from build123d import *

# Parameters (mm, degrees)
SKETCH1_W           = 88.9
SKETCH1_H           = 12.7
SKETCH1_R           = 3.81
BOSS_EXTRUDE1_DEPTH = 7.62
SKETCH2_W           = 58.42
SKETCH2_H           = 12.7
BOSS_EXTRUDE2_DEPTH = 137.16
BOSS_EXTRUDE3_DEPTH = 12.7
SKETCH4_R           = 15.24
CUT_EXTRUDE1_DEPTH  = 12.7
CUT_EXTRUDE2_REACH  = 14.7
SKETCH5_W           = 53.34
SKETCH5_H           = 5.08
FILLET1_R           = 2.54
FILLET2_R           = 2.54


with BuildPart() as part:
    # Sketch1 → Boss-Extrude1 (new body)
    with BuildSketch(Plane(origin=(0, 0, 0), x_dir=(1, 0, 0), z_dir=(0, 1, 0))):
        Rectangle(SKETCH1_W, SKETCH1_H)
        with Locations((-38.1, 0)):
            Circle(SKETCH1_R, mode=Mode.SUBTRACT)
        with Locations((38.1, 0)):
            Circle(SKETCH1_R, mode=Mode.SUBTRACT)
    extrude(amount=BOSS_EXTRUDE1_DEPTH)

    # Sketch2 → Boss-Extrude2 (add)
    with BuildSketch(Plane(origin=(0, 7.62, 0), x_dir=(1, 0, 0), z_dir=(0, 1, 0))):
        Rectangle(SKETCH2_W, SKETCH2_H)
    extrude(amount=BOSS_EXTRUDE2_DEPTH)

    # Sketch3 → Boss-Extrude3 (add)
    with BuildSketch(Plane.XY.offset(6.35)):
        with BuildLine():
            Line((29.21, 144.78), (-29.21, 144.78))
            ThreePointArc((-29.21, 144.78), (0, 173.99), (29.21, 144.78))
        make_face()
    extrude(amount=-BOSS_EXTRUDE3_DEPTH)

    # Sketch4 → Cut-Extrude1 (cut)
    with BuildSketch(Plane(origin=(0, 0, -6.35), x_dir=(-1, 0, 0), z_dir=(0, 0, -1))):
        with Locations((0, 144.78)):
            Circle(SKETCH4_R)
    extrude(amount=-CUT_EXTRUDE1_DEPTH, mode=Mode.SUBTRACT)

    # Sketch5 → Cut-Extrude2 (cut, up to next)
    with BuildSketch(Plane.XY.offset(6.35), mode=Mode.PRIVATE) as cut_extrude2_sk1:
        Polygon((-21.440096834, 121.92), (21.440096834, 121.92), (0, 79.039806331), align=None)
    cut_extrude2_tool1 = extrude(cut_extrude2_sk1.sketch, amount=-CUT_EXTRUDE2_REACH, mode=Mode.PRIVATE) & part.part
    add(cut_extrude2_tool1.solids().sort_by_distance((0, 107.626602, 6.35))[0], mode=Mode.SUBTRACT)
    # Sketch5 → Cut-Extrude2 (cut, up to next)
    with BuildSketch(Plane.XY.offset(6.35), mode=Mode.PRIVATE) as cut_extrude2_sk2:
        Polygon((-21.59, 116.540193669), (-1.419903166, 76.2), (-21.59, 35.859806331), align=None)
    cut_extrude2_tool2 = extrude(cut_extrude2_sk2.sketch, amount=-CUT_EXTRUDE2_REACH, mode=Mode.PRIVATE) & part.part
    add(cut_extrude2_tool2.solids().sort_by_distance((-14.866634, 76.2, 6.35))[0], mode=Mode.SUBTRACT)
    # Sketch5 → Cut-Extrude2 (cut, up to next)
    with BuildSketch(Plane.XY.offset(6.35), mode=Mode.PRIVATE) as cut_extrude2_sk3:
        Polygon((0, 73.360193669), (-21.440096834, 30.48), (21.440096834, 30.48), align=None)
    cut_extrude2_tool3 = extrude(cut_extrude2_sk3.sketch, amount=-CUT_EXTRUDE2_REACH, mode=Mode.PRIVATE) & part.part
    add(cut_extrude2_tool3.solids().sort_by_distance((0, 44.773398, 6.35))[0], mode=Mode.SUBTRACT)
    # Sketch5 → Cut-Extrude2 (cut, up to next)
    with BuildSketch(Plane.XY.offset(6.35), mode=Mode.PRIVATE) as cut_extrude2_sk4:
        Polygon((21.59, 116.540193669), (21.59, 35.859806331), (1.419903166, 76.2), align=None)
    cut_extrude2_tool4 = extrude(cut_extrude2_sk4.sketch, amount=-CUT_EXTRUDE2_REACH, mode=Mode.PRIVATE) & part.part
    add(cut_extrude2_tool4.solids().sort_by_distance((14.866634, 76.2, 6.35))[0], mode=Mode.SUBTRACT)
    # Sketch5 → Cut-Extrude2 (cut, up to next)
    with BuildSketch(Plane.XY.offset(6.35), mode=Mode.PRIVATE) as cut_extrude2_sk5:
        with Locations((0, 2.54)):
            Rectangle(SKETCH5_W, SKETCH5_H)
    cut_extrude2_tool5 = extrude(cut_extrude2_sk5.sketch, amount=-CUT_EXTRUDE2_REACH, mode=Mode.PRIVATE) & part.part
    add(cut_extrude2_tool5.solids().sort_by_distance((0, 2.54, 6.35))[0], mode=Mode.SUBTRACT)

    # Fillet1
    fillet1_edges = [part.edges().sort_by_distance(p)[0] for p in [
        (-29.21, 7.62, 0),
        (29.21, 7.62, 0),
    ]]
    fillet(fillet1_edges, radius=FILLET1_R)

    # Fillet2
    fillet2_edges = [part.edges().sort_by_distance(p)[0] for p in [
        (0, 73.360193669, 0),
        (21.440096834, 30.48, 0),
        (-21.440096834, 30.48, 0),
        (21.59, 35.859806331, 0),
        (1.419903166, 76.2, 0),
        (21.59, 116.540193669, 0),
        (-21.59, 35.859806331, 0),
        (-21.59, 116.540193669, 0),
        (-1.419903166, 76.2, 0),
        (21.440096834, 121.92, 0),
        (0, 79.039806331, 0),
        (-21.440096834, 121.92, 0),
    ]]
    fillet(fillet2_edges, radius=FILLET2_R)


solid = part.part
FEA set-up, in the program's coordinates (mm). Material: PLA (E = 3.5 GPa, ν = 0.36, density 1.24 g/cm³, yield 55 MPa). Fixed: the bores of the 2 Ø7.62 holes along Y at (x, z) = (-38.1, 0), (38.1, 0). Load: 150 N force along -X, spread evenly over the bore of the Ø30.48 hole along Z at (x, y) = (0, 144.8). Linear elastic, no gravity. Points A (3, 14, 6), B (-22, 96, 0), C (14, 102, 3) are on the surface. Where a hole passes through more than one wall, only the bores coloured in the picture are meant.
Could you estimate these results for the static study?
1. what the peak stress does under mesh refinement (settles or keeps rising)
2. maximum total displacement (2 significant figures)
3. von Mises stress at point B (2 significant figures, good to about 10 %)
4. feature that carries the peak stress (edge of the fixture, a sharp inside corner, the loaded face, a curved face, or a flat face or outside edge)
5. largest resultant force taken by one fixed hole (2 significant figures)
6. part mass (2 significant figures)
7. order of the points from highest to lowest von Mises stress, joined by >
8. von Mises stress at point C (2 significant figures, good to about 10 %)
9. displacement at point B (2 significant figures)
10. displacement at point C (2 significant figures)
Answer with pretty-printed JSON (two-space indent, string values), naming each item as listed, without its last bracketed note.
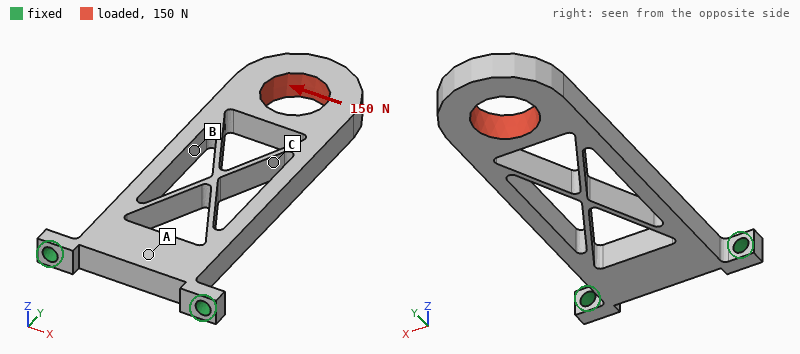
{
  "what the peak stress does under mesh refinement": "keeps rising",
  "maximum total displacement": "0.88 mm",
  "von Mises stress at point B": "3.5 MPa",
  "feature that carries the peak stress": "edge of the fixture",
  "largest resultant force taken by one fixed hole": "360 N",
  "part mass": "88 g",
  "order of the points from highest to lowest von Mises stress, joined by >": "C > B > A",
  "von Mises stress at point C": "5.8 MPa",
  "displacement at point B": "0.47 mm",
  "displacement at point C": "0.52 mm"
}
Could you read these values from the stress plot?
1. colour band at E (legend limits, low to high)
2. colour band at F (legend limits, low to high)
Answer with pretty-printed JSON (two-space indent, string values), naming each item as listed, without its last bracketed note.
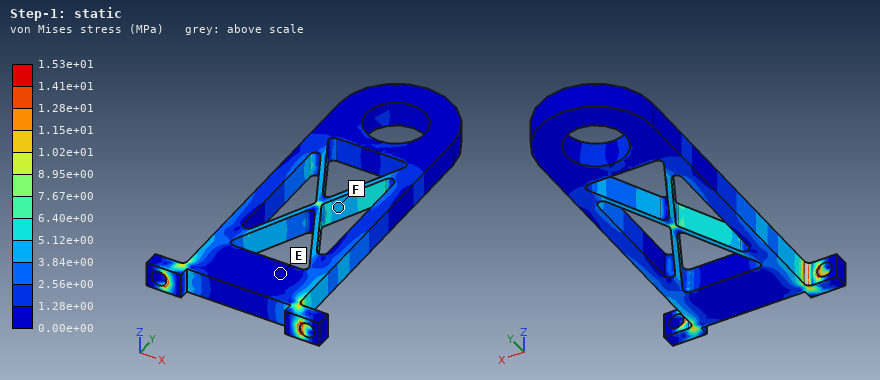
{
  "colour band at E": "0.00e+00 to 1.28e+00 MPa",
  "colour band at F": "3.84e+00 to 5.12e+00 MPa"
}
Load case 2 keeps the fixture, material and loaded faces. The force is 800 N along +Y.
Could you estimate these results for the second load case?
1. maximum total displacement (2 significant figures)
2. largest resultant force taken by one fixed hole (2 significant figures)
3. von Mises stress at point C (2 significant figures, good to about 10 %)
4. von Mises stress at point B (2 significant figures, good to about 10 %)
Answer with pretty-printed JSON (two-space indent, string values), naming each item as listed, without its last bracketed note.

{
  "maximum total displacement": "0.20 mm",
  "largest resultant force taken by one fixed hole": "460 N",
  "von Mises stress at point C": "1.4 MPa",
  "von Mises stress at point B": "4.5 MPa"
}
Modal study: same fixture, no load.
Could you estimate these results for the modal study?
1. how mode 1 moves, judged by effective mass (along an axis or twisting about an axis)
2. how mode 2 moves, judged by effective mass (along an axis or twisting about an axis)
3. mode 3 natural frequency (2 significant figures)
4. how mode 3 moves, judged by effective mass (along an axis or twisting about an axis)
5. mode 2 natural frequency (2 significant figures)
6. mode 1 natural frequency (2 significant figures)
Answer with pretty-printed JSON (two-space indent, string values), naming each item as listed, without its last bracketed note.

{
  "how mode 1 moves, judged by effective mass": "along Z",
  "how mode 2 moves, judged by effective mass": "along X",
  "mode 3 natural frequency": "370 Hz",
  "how mode 3 moves, judged by effective mass": "twisting about Y",
  "mode 2 natural frequency": "360 Hz",
  "mode 1 natural frequency": "73 Hz"
}
